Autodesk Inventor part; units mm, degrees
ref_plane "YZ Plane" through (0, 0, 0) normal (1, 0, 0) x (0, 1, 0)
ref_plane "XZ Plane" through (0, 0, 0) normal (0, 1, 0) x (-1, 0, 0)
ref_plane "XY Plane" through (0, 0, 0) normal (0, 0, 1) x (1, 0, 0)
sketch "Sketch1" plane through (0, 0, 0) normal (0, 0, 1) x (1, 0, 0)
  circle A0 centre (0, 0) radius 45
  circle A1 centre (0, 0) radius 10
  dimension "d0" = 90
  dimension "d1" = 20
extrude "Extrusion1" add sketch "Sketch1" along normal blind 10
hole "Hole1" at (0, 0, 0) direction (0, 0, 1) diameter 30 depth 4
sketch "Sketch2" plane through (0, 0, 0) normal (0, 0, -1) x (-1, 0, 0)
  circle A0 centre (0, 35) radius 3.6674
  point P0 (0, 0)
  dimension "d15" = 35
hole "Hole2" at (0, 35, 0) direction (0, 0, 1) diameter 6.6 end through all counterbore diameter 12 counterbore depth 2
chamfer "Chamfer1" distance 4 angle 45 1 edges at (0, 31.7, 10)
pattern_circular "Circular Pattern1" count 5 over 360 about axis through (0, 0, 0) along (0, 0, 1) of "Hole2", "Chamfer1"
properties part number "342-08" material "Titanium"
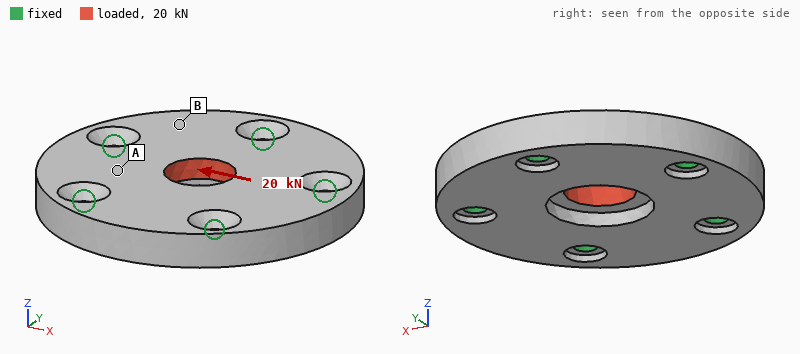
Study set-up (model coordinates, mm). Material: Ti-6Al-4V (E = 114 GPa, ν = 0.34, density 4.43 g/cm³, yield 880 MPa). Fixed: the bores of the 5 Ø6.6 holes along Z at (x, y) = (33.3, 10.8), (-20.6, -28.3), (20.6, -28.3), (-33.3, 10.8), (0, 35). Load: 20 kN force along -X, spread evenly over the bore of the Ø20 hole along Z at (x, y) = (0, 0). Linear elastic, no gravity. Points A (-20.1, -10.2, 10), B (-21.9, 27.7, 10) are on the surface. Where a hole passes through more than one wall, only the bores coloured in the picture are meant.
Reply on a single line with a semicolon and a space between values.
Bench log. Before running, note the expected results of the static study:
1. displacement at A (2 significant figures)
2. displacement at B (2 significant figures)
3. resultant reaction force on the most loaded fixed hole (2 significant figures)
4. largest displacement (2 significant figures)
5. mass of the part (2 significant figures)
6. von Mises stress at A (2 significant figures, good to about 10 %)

6.5 µm; 3.6 µm; 5.3 kN; 13 µm; 240 g; 24 MPa
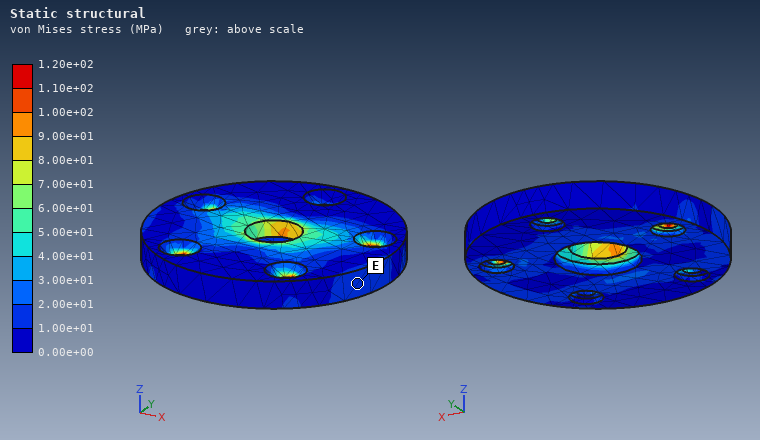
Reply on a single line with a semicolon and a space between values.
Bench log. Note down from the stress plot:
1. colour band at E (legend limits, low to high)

1.00e+01 to 2.00e+01 MPa
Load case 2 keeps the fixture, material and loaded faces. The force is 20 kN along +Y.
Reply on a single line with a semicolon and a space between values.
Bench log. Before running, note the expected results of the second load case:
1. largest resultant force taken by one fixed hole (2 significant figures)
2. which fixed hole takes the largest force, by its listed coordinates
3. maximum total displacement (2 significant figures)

5.5 kN; (0, 35); 13 µm
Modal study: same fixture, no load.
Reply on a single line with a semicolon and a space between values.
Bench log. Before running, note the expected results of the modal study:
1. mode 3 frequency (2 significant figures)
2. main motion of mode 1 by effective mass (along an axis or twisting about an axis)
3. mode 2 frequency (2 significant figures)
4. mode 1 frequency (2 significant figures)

13 kHz; along Z; 13 kHz; 12 kHz
